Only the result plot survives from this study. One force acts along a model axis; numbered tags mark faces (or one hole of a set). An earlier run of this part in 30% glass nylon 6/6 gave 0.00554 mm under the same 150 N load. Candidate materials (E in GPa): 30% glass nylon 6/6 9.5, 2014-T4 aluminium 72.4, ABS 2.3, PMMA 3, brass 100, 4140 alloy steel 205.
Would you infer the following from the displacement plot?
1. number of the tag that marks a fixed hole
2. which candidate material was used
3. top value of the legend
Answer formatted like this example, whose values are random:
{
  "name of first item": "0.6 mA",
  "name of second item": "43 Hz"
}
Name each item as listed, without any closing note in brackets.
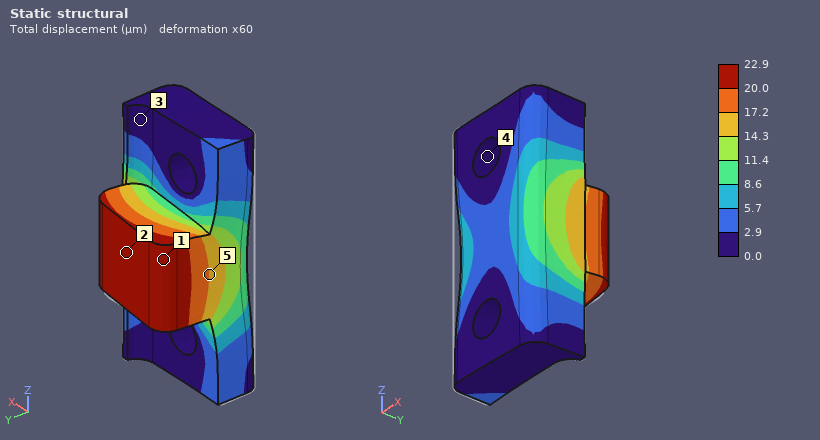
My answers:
{
  "number of the tag that marks a fixed hole": "4",
  "which candidate material was used": "ABS",
  "top value of the legend": "22.9 µm"
}
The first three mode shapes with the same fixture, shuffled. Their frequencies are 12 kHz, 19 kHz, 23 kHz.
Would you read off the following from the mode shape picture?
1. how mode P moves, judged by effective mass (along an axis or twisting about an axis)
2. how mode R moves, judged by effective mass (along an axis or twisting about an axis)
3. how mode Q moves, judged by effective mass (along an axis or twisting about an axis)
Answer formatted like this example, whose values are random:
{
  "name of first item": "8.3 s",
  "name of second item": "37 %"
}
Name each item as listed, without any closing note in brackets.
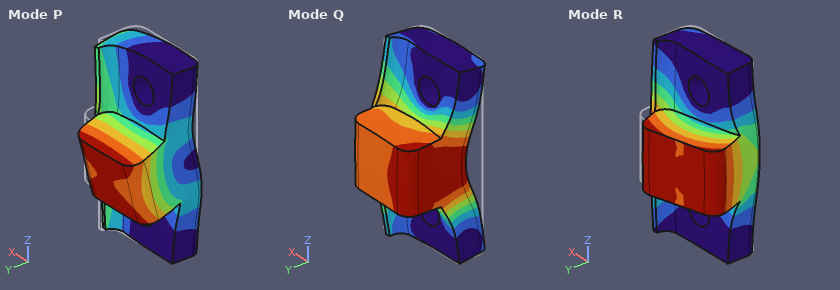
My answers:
{
  "how mode P moves, judged by effective mass": "along Z",
  "how mode R moves, judged by effective mass": "along X",
  "how mode Q moves, judged by effective mass": "along Y"
}
